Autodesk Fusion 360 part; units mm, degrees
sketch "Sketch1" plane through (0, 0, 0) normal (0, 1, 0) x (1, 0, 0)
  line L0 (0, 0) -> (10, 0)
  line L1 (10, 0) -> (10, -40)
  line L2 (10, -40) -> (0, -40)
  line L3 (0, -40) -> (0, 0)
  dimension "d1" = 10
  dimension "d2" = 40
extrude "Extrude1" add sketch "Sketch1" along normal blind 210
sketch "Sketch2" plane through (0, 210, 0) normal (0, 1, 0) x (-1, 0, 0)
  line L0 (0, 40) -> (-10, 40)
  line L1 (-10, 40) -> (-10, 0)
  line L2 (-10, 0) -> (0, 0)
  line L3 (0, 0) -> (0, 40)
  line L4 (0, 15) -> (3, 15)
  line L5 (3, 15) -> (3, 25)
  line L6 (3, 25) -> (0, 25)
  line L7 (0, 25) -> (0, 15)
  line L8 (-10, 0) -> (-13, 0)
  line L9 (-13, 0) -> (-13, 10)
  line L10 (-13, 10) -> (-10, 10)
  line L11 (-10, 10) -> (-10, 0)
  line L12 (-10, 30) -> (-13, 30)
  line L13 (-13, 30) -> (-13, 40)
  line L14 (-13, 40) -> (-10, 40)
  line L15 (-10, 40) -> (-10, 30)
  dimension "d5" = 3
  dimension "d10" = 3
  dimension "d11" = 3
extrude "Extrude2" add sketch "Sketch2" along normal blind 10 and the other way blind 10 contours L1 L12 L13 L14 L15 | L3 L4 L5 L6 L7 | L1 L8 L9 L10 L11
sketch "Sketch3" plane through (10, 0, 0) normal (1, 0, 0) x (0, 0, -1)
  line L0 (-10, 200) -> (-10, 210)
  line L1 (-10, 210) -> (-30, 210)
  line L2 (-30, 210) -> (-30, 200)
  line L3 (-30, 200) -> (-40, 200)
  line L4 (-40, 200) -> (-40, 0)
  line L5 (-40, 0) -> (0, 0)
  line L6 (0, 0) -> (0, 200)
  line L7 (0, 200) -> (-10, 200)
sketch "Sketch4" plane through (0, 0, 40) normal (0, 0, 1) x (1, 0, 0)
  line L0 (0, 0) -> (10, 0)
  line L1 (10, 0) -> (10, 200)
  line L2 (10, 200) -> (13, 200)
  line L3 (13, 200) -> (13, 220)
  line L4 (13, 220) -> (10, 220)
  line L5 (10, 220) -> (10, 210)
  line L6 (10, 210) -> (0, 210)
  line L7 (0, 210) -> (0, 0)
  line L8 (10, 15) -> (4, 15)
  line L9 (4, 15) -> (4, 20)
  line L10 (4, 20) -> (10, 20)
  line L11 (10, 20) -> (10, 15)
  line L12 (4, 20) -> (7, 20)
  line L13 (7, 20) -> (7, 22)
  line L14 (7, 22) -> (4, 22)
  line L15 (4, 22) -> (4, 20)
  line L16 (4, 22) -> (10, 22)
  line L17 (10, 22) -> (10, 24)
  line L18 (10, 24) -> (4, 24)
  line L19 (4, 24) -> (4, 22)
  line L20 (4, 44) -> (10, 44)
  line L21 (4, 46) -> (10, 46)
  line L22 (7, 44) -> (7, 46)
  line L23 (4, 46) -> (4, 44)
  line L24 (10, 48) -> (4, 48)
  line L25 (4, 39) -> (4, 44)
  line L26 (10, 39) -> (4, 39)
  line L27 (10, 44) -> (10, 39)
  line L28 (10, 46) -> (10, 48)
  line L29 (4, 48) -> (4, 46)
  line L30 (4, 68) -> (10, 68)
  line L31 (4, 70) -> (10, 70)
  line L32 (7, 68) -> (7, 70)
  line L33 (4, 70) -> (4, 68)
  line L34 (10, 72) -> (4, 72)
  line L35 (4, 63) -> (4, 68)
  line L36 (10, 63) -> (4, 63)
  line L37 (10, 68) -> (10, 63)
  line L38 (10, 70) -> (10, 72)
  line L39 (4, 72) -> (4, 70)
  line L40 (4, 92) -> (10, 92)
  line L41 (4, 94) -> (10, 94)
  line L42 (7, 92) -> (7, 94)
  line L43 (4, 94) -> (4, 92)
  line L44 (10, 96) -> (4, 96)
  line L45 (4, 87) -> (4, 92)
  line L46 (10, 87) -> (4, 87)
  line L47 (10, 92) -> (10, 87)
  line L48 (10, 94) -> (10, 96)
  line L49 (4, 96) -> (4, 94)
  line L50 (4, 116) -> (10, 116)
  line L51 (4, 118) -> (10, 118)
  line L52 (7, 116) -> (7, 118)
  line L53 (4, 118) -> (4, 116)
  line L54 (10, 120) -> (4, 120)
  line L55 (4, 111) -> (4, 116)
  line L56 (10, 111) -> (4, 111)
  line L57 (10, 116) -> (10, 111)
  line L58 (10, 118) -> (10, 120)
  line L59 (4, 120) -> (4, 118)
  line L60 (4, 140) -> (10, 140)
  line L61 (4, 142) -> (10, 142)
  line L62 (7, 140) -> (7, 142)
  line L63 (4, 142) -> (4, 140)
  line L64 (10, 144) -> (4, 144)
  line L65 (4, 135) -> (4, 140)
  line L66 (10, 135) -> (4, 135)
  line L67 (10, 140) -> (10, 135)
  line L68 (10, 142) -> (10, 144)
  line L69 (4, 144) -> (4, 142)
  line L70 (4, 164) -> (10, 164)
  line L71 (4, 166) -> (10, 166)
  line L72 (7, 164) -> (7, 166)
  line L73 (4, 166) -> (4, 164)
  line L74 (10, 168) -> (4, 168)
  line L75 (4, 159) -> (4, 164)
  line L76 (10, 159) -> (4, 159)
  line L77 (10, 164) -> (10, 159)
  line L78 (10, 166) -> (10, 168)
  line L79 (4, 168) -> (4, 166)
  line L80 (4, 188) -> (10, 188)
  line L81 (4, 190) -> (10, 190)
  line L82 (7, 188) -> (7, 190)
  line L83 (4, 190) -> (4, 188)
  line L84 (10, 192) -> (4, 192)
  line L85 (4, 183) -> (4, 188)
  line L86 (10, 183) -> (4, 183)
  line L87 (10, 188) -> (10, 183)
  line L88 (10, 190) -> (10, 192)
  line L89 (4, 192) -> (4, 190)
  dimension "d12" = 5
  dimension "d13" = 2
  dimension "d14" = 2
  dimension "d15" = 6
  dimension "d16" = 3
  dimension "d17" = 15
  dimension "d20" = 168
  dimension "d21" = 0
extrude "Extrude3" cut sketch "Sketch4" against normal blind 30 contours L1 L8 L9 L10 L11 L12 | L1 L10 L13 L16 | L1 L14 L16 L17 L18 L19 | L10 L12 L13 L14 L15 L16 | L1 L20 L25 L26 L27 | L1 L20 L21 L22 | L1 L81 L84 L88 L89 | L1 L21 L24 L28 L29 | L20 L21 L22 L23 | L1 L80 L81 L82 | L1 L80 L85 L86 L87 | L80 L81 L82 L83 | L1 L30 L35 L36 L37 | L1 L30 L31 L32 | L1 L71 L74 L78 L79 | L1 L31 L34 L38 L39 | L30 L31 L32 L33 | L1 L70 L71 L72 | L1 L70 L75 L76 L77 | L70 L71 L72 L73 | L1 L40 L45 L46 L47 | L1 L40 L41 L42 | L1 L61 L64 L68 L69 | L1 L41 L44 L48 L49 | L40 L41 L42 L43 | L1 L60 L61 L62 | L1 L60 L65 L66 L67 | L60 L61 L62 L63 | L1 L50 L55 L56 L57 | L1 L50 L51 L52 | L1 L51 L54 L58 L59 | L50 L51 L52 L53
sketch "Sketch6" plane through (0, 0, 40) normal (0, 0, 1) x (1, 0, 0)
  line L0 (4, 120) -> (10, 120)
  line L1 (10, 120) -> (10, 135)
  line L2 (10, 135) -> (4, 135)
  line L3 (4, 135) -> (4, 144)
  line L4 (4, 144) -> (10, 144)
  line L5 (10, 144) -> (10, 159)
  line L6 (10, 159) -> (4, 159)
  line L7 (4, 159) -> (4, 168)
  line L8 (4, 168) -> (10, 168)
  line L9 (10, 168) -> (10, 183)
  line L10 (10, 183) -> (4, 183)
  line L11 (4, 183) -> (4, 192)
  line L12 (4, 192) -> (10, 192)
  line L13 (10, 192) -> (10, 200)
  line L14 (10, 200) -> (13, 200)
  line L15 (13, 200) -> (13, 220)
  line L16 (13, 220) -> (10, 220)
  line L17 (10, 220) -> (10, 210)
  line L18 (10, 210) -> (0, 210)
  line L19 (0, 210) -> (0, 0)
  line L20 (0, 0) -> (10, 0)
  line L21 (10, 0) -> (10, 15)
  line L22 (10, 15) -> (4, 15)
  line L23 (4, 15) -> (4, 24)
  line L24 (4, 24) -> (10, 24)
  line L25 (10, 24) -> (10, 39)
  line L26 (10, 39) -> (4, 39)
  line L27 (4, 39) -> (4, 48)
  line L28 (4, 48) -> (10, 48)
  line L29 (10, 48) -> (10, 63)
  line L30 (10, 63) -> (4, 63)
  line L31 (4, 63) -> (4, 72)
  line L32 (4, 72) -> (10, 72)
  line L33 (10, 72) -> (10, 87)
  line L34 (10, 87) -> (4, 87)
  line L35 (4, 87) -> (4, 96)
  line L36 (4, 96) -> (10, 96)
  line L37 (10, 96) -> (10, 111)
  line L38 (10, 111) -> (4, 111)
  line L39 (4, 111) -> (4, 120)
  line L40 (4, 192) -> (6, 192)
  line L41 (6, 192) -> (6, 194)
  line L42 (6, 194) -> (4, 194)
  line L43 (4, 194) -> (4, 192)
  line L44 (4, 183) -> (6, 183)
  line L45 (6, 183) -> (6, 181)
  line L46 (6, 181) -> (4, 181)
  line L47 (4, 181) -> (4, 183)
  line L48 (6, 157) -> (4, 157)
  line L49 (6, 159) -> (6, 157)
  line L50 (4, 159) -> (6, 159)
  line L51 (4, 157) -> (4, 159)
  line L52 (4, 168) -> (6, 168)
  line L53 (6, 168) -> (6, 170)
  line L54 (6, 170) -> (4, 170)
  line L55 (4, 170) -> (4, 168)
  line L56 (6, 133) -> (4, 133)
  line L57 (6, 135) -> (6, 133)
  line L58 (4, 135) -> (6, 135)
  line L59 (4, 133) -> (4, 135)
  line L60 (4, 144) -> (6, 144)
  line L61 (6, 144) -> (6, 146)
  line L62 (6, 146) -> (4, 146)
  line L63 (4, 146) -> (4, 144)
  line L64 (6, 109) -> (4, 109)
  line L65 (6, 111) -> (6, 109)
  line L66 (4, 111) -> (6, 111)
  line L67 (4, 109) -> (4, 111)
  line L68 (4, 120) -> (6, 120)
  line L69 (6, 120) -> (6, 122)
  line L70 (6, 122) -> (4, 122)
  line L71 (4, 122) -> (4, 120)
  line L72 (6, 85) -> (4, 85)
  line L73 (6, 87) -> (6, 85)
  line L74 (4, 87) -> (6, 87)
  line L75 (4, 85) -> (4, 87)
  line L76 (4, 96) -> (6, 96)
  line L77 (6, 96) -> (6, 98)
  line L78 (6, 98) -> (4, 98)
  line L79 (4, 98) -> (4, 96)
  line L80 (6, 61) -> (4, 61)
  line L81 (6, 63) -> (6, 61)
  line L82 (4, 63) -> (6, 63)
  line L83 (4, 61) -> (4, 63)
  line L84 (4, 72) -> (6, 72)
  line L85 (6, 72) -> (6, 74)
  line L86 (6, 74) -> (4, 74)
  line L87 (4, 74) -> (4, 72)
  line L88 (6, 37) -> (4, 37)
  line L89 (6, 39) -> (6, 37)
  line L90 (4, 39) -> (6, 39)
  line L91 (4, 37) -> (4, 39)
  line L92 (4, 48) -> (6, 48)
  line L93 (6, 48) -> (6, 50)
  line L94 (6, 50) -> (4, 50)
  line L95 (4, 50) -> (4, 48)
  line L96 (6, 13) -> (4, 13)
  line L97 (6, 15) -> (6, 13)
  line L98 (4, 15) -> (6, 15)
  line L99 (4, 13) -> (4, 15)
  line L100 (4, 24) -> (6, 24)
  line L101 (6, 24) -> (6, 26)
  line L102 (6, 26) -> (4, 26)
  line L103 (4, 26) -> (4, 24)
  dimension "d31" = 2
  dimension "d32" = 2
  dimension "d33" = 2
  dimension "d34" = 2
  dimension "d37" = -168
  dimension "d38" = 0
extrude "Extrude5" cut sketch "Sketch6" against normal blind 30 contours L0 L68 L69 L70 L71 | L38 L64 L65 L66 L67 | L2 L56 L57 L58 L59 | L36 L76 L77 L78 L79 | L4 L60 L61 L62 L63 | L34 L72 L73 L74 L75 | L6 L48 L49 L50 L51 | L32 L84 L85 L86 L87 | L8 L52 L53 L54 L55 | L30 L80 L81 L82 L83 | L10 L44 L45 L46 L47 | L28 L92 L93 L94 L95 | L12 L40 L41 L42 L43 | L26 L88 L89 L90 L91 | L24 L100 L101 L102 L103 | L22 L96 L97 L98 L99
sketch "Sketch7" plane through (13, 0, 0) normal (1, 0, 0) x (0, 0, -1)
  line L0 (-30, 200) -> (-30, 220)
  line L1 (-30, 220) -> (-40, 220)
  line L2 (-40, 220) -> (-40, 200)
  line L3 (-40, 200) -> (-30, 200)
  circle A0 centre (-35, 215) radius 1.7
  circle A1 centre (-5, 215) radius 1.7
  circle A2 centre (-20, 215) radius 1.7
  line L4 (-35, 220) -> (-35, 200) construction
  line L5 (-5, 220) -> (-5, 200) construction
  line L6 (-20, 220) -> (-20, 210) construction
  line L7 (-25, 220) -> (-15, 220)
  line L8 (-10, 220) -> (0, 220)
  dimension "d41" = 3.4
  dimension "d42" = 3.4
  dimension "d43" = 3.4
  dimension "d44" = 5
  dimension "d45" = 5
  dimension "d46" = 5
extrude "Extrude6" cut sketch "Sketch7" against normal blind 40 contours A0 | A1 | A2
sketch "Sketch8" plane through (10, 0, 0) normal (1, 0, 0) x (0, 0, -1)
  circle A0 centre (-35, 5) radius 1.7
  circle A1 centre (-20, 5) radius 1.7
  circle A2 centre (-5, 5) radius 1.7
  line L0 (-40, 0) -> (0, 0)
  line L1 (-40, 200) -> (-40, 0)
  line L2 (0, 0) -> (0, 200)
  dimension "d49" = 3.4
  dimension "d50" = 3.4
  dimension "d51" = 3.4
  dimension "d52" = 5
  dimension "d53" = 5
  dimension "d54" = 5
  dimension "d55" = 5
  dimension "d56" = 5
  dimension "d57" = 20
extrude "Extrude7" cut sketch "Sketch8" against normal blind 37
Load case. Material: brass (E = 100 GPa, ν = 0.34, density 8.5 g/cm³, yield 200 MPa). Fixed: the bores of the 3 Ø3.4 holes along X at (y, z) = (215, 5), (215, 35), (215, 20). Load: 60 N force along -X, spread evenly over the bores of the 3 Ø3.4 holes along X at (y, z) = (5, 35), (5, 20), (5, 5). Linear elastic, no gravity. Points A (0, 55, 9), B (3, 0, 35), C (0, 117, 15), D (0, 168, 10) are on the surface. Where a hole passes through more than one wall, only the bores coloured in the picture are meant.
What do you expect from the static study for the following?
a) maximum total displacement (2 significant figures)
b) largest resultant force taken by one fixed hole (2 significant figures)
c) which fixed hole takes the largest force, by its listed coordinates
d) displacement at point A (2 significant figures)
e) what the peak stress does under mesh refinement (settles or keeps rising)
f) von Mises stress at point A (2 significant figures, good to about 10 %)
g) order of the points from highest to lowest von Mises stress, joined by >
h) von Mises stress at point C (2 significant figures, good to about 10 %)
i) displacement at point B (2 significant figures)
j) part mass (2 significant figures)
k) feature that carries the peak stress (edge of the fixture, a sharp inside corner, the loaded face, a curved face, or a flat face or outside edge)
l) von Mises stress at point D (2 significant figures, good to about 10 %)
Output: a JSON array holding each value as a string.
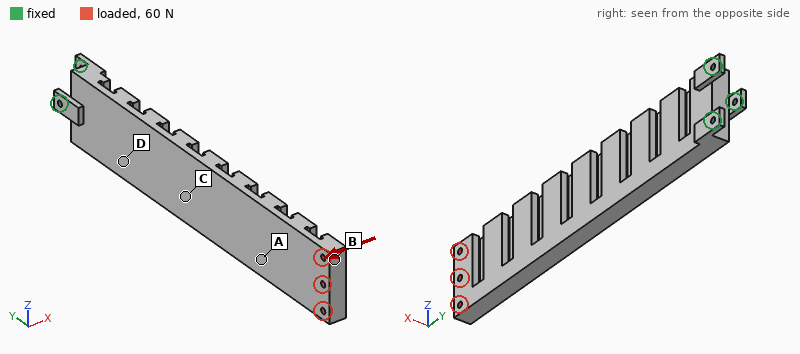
["1.4 mm", "950 N", "(215, 20)", "0.83 mm", "keeps rising", "9.0 MPa", "D > C > A > B", "20 MPa", "1.4 mm", "600 g", "edge of the fixture", "33 MPa"]
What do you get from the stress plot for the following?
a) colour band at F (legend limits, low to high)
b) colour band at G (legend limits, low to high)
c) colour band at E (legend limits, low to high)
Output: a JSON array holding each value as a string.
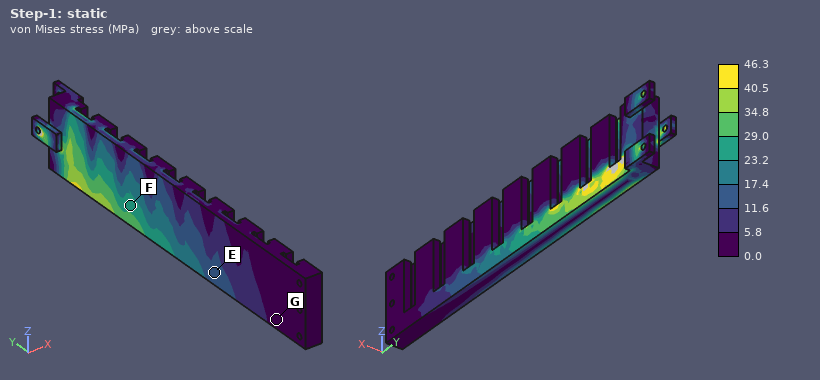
["23.2 to 29.0 MPa", "0.0 to 5.8 MPa", "11.6 to 17.4 MPa"]
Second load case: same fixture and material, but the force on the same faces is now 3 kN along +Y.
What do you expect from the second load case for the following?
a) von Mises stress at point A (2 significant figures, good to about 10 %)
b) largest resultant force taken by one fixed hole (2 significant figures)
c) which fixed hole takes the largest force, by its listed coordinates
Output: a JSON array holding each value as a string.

["5.5 MPa", "1.5 kN", "(215, 20)"]
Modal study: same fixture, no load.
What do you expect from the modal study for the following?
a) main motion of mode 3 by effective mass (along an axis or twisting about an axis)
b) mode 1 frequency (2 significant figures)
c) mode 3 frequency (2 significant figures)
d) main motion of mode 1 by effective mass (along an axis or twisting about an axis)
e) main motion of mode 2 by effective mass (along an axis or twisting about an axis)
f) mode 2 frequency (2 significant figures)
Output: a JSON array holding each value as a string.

["along X", "87 Hz", "530 Hz", "along X", "along Z", "320 Hz"]
